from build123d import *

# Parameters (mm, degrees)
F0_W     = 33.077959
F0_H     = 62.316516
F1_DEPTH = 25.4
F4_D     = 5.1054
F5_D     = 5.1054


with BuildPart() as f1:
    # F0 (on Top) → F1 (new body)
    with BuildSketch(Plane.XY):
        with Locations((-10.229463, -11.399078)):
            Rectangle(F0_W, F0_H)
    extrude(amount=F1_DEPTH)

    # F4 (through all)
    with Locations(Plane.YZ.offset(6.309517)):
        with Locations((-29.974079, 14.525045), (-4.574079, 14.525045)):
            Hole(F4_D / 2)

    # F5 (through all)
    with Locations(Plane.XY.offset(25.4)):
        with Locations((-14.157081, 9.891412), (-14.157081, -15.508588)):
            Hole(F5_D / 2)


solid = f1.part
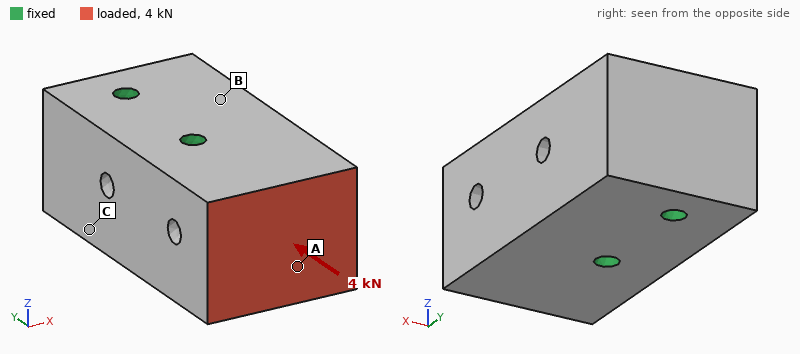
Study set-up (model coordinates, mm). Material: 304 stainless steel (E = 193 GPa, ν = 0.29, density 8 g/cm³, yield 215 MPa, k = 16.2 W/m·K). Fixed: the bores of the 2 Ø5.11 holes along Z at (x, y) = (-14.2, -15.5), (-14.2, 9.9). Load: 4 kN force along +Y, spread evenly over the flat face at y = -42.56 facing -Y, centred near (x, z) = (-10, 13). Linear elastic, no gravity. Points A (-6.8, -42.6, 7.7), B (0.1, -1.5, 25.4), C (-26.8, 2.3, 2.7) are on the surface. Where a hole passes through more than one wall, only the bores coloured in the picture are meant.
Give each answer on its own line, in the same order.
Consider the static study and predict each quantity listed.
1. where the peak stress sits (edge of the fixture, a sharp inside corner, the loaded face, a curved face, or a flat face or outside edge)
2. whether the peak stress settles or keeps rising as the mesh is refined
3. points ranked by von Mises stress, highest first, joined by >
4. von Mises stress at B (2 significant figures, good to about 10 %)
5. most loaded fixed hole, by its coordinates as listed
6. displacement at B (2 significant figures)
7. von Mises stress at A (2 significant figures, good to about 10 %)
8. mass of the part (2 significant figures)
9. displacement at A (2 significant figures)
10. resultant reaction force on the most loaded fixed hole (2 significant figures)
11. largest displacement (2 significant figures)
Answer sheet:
edge of the fixture
keeps rising
A > B > C
2.7 MPa
(-14.2, -15.5)
0.32 µm
4.9 MPa
400 g
1.2 µm
3.2 kN
1.5 µm
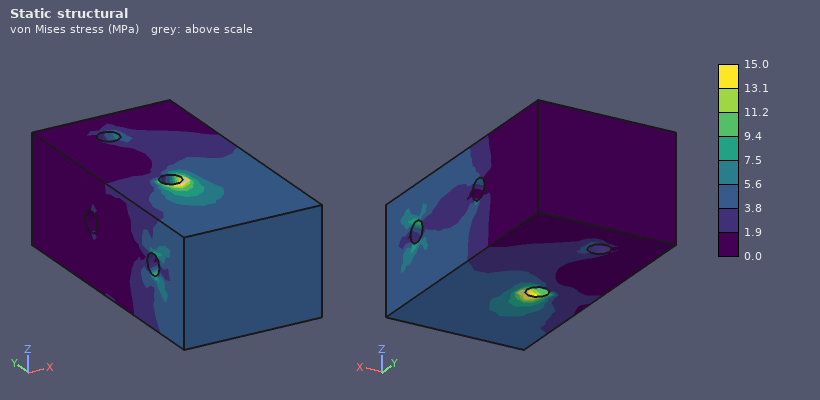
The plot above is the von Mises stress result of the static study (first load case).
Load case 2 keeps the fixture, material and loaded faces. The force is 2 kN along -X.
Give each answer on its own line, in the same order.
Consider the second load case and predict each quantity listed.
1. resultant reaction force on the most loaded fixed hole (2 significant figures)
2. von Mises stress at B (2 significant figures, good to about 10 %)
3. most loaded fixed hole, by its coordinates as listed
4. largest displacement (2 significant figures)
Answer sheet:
3.6 kN
5.6 MPa
(-14.2, -15.5)
4.6 µm
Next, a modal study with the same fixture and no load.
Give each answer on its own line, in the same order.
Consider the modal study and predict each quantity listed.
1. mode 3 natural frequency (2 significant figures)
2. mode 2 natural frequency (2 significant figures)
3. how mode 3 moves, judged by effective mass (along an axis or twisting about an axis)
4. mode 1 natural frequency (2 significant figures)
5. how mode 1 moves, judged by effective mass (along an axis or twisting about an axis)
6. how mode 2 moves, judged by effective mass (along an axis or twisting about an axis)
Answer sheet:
20 kHz
15 kHz
twisting about Y
13 kHz
along X
along Z
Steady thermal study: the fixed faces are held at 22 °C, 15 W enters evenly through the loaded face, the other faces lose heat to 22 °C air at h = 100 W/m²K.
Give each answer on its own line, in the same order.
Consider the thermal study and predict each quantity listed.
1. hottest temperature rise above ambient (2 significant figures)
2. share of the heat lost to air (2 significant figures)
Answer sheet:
28 K
38 %
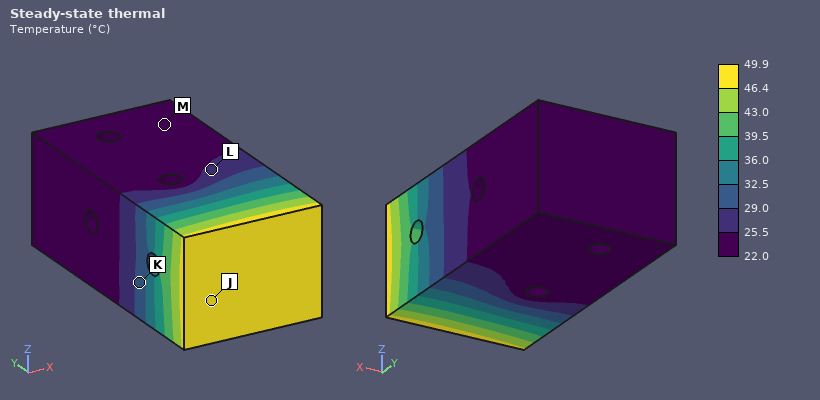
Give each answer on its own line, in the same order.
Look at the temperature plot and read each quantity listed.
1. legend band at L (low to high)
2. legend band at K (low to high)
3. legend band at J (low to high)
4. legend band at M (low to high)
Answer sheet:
25.5 to 29.0 °C
29.0 to 32.5 °C
46.4 to 49.9 °C
22.0 to 25.5 °C
